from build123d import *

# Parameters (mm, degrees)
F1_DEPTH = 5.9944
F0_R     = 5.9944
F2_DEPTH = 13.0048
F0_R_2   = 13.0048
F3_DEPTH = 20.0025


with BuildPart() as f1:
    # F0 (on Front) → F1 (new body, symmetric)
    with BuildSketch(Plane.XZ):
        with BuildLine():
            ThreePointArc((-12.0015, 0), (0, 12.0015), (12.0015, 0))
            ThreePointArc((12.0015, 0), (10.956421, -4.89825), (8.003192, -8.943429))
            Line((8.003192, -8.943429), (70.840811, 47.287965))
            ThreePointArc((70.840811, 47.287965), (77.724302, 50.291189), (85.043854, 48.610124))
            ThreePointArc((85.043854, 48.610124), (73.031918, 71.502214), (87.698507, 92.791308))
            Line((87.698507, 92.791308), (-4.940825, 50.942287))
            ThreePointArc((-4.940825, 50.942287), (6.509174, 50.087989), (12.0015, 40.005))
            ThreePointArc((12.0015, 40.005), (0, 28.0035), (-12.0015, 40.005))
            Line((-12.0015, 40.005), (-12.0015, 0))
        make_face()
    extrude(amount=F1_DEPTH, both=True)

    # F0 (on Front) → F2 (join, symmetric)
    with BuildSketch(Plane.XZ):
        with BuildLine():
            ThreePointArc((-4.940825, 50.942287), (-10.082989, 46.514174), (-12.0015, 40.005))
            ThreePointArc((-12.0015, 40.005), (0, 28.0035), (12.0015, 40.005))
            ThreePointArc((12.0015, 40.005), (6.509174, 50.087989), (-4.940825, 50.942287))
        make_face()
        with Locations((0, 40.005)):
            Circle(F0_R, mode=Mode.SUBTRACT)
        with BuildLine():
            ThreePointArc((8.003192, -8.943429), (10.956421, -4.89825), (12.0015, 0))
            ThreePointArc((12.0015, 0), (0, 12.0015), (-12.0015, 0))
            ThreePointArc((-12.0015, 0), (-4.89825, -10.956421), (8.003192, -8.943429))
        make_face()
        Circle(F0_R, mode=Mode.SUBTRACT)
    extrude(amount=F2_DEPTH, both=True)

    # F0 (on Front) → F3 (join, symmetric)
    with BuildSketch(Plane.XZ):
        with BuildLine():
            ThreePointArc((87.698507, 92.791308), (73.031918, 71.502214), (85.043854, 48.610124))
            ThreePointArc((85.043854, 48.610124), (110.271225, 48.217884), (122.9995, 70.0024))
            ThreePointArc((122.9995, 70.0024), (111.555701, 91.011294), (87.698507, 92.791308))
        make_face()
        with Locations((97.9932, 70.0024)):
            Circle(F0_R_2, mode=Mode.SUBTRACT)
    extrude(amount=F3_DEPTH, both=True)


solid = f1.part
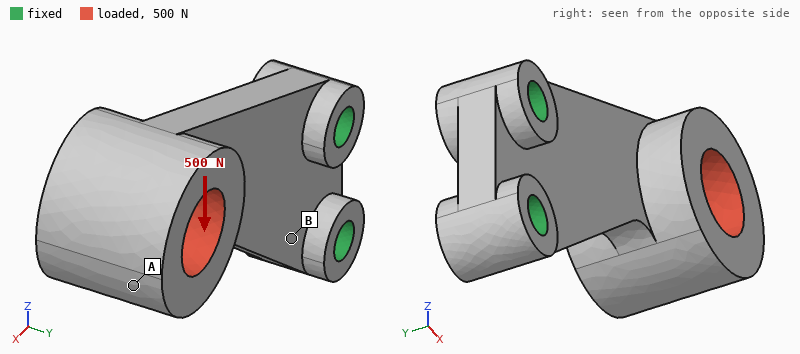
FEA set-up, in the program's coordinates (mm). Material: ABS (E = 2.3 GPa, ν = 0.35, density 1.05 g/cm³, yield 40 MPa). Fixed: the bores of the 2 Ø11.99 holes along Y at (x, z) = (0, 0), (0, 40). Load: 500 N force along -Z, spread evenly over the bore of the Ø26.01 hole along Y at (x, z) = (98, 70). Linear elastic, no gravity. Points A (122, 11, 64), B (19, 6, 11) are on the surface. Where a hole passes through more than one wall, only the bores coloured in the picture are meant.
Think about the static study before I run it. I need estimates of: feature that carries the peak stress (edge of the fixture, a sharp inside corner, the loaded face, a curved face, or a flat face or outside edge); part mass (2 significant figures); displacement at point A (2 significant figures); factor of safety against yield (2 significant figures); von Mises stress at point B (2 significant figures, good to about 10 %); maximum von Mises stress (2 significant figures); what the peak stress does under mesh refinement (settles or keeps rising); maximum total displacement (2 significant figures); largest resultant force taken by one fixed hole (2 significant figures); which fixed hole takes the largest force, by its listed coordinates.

a curved face
130 g
1.2 mm
3.7
5.5 MPa
11 MPa
settles
1.3 mm
1.2 kN
(0, 0)
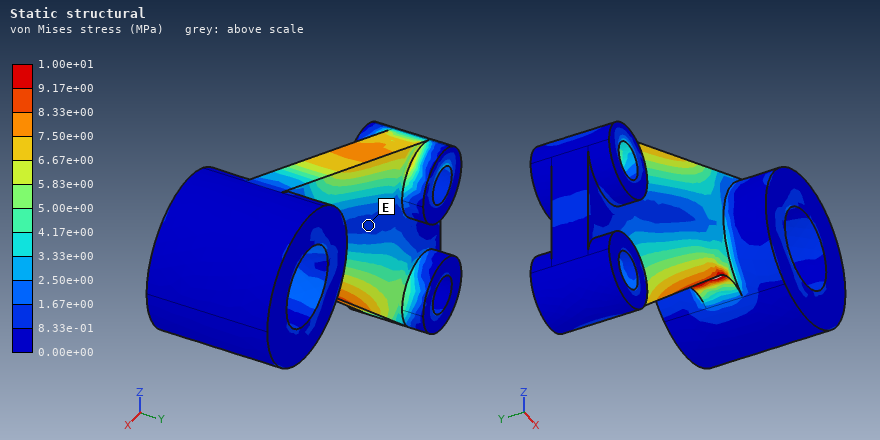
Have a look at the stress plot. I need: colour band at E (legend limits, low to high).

8.33e-01 to 1.67e+00 MPa
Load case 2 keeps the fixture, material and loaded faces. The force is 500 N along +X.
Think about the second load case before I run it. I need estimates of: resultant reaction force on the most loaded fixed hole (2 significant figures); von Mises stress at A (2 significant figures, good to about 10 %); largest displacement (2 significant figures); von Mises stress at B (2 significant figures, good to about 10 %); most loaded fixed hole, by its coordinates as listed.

790 N
0.38 MPa
0.44 mm
1.7 MPa
(0, 40)
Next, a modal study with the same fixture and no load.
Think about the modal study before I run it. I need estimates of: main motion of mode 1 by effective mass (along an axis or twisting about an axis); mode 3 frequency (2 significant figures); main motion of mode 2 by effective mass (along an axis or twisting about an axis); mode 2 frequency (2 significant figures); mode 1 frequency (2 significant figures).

along Y
530 Hz
along Z
430 Hz
130 Hz
